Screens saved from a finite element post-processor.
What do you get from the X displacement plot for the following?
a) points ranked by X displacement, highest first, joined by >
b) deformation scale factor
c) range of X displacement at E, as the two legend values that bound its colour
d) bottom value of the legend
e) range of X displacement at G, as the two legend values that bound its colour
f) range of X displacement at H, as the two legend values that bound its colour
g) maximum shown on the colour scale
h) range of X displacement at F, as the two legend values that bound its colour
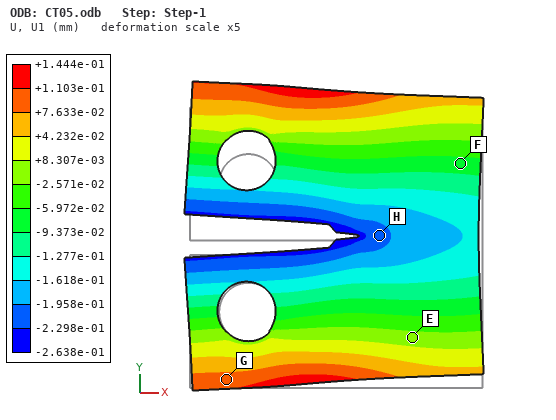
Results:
G > E > F > H
5
-2.571e-02 to +8.307e-03 mm
-2.638e-01 mm
+7.633e-02 to +1.103e-01 mm
-2.298e-01 to -1.958e-01 mm
+1.444e-01 mm
-9.373e-02 to -5.972e-02 mm
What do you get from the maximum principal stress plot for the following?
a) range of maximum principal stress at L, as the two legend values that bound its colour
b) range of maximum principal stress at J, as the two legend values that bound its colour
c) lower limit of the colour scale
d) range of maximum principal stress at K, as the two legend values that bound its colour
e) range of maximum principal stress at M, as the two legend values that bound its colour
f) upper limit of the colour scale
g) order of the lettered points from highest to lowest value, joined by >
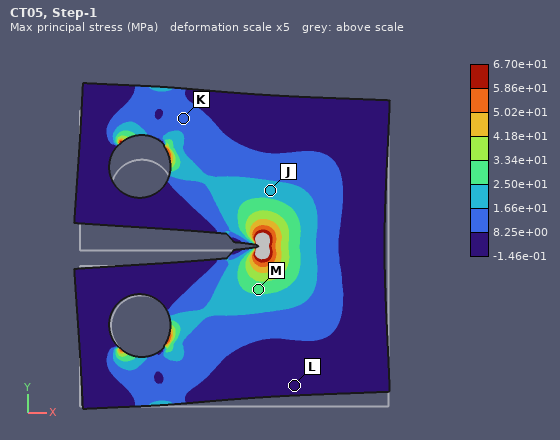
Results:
-1.46e-01 to 8.25e+00 MPa
1.66e+01 to 2.50e+01 MPa
-1.46e-01 MPa
8.25e+00 to 1.66e+01 MPa
2.50e+01 to 3.34e+01 MPa
6.70e+01 MPa
M > J > K > L
